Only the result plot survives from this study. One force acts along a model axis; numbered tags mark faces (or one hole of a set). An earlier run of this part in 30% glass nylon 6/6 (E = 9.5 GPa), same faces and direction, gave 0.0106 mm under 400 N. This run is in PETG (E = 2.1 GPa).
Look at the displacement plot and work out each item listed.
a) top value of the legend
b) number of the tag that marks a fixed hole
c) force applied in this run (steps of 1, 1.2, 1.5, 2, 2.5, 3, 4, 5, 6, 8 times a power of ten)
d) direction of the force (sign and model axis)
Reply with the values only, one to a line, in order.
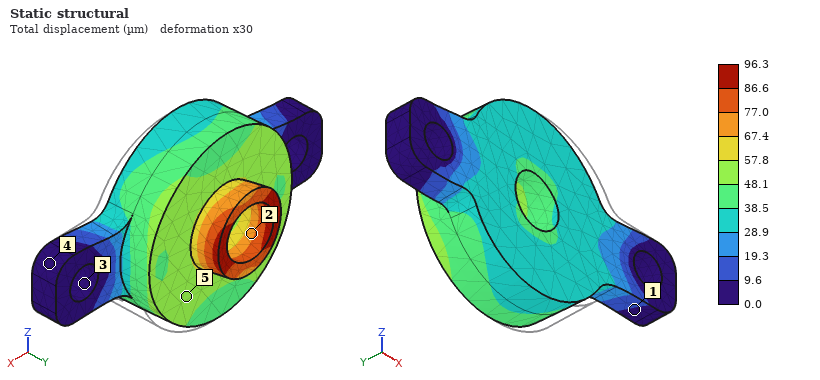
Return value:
96.3 µm
3
800 N
-X
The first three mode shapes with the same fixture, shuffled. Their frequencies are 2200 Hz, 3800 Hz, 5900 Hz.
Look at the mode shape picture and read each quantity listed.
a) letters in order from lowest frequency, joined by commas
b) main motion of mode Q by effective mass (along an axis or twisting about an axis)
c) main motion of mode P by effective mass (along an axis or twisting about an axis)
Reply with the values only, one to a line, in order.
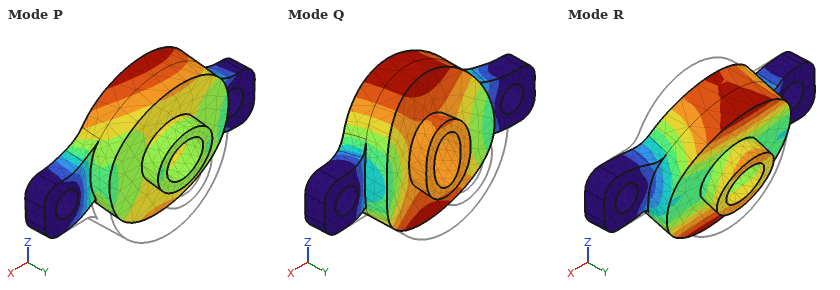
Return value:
R, Q, P
along Y
along Z
